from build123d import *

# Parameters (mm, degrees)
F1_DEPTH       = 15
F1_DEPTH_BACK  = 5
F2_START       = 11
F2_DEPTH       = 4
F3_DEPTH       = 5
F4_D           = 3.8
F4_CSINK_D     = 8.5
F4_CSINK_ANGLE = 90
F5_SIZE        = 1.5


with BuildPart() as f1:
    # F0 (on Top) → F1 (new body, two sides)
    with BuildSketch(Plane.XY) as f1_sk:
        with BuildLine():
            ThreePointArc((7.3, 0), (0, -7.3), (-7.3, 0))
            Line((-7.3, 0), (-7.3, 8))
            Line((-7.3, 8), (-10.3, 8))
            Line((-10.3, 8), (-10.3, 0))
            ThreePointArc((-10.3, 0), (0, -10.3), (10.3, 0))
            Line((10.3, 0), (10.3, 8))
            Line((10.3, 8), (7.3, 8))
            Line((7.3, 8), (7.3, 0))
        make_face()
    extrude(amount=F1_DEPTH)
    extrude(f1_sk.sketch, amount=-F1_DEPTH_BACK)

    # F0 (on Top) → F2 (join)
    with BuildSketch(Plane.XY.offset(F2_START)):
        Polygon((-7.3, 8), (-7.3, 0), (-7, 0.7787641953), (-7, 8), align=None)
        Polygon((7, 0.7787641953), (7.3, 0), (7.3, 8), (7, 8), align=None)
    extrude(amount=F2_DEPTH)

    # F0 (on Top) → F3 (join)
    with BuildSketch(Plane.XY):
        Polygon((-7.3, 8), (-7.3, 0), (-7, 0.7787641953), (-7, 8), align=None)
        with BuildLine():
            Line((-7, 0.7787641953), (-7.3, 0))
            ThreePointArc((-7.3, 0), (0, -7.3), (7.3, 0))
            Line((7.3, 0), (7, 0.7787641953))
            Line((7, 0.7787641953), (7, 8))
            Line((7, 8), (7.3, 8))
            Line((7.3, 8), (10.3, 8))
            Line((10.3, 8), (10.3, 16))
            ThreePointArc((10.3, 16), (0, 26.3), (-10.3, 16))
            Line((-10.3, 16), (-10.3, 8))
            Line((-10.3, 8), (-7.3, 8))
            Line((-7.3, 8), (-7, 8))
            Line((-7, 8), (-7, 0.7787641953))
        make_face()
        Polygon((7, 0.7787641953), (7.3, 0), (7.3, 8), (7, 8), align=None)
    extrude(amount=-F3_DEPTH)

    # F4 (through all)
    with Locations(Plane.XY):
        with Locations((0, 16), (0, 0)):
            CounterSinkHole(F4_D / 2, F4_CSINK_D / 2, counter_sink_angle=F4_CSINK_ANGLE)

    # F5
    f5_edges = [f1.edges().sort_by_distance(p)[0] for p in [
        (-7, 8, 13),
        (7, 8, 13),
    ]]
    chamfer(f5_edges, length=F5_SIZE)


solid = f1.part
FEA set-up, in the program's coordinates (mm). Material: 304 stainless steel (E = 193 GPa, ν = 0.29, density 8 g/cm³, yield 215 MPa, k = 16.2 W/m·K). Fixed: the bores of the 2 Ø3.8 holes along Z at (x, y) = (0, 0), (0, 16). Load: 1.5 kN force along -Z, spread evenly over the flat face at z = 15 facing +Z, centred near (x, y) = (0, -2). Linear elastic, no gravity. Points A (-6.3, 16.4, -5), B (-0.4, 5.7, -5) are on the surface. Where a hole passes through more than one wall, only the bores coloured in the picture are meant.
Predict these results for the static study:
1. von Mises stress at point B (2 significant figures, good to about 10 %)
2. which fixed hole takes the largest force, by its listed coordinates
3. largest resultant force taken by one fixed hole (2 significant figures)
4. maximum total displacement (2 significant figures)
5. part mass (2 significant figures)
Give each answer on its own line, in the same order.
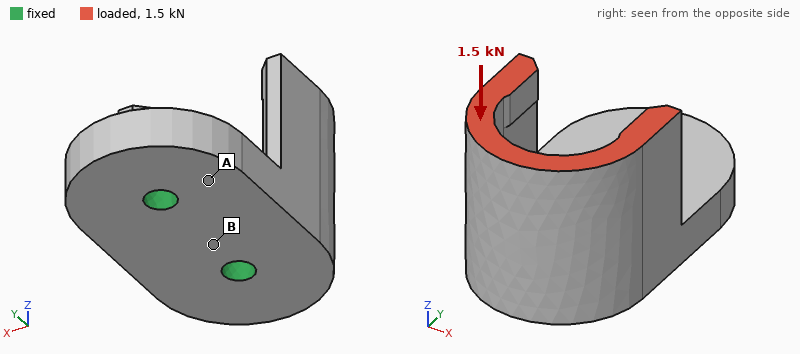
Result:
23 MPa
(0, 0)
1.5 kN
8.3 µm
41 g
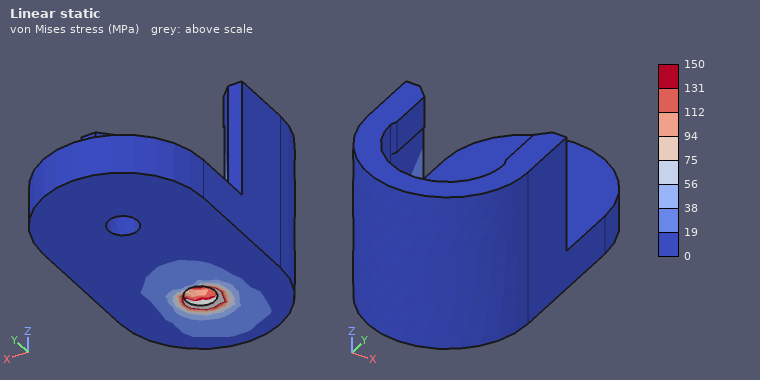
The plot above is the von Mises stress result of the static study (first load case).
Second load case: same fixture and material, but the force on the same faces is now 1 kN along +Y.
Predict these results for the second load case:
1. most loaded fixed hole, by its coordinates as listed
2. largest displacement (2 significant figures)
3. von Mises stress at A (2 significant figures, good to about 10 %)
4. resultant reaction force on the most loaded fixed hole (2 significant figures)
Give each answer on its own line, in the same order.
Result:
(0, 16)
30 µm
23 MPa
1.4 kN
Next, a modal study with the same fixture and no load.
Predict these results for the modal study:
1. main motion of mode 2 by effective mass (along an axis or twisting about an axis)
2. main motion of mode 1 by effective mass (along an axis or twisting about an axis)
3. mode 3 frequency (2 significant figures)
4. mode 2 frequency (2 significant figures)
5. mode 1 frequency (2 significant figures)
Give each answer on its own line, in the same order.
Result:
along Y
along X
14 kHz
11 kHz
6700 Hz
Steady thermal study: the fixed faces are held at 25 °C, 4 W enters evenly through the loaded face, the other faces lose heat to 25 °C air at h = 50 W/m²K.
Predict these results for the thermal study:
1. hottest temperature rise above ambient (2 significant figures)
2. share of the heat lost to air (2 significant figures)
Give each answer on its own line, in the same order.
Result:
32 K
43 %
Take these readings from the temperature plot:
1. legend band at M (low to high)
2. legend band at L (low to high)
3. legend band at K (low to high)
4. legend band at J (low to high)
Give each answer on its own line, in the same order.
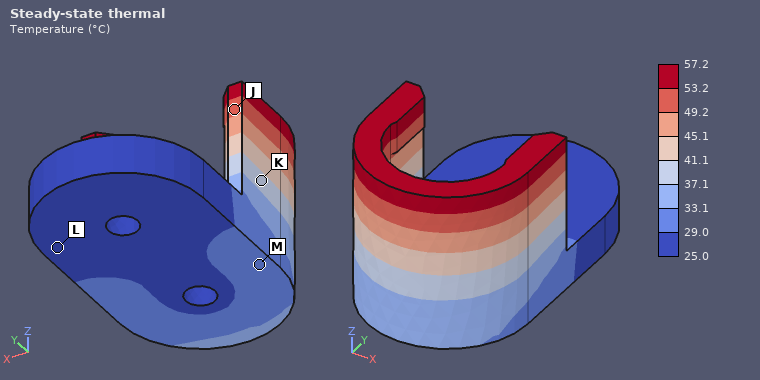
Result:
29.0 to 33.1 °C
25.0 to 29.0 °C
37.1 to 41.1 °C
49.2 to 53.2 °C
